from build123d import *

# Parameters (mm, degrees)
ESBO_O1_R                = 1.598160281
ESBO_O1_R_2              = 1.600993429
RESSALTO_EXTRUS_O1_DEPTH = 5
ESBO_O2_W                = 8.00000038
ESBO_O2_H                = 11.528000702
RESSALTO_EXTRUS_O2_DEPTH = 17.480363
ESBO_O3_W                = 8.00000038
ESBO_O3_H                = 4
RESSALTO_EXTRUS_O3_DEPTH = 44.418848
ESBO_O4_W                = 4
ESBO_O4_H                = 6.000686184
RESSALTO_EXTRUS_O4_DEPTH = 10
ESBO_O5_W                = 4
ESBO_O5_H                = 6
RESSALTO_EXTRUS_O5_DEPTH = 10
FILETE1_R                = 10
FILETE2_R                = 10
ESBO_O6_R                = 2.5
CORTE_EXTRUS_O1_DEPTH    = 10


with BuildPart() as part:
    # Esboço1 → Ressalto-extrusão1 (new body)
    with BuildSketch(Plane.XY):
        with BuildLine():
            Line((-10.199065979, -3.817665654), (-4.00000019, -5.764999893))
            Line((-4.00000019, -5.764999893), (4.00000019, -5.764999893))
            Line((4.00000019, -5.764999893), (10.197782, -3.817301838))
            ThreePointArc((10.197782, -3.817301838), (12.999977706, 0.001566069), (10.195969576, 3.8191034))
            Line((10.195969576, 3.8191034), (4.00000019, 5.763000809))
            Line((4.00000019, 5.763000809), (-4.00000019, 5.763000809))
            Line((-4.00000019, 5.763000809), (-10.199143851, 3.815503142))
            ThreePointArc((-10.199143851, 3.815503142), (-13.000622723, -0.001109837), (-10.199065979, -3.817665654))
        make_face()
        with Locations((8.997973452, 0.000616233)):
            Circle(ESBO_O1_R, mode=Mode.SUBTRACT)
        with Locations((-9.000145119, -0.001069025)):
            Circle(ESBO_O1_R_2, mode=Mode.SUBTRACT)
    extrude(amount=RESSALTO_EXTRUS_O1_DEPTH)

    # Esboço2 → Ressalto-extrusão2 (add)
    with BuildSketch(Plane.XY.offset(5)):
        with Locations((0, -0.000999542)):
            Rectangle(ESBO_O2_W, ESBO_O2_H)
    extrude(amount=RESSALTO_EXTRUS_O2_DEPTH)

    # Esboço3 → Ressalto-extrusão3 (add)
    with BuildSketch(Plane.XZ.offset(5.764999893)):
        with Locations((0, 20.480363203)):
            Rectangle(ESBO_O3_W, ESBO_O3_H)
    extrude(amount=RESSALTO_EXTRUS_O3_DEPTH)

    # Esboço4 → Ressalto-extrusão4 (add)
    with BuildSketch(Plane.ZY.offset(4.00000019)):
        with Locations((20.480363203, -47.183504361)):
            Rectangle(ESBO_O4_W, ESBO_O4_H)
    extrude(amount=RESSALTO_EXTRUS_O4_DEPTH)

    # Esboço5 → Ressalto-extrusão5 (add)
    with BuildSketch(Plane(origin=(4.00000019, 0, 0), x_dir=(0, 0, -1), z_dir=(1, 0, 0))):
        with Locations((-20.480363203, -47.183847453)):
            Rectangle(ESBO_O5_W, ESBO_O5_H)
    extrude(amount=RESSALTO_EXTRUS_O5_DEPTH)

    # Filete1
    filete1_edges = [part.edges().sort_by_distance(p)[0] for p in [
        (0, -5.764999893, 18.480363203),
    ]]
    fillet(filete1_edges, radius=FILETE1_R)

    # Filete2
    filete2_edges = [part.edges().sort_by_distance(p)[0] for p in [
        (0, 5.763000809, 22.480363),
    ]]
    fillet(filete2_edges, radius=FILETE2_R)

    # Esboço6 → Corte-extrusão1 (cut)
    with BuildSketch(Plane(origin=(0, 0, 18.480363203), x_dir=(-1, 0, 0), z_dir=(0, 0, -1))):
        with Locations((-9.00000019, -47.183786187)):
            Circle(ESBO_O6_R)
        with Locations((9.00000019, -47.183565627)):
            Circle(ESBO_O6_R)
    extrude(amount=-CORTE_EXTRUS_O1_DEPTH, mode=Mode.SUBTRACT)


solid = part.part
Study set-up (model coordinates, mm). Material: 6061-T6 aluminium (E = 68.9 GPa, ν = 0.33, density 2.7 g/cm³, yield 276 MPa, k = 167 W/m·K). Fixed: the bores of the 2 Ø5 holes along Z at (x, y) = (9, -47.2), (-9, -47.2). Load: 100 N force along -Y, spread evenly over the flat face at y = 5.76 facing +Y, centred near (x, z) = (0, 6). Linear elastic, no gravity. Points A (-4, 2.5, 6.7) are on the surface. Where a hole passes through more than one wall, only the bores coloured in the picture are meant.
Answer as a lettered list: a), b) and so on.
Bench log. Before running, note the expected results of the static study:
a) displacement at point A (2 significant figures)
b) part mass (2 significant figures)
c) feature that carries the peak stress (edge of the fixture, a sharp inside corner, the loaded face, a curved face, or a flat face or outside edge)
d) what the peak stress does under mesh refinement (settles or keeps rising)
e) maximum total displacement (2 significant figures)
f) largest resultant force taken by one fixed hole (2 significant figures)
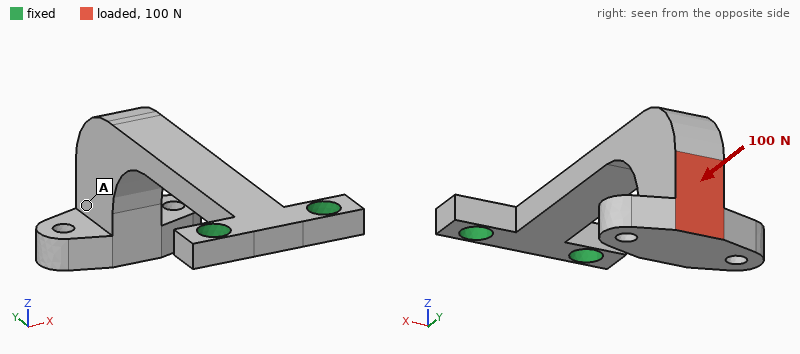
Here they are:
a) 0.65 mm
b) 12 g
c) a sharp inside corner
d) keeps rising
e) 0.76 mm
f) 52 N
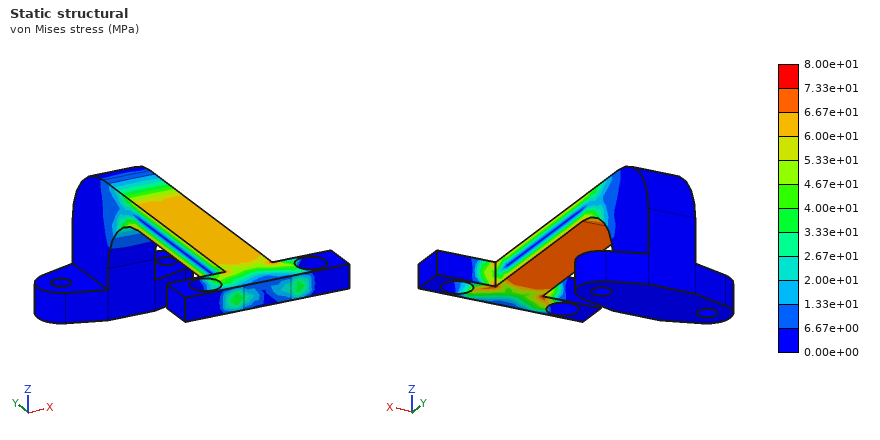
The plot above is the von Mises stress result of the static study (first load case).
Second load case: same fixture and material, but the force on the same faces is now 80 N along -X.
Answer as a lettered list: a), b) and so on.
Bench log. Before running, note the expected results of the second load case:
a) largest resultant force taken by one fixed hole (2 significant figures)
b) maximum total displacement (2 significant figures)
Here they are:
a) 360 N
b) 0.59 mm
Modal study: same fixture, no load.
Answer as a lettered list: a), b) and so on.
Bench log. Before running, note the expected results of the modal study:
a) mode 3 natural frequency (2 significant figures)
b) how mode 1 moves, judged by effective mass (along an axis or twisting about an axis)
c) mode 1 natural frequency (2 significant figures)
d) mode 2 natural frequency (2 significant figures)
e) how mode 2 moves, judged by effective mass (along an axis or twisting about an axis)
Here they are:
a) 2500 Hz
b) along Z
c) 470 Hz
d) 840 Hz
e) along X
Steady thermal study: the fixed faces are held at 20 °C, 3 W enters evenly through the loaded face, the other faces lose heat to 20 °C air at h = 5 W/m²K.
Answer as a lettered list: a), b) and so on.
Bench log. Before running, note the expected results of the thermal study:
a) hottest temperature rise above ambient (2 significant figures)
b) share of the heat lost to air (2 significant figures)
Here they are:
a) 25 K
b) 7.1 %
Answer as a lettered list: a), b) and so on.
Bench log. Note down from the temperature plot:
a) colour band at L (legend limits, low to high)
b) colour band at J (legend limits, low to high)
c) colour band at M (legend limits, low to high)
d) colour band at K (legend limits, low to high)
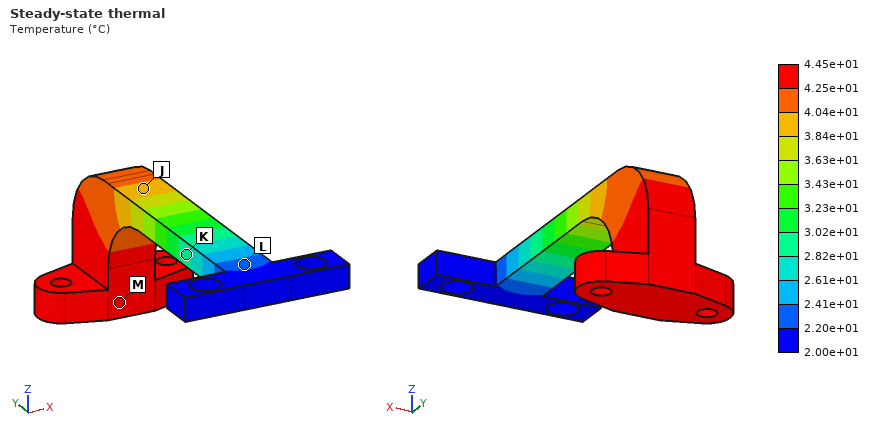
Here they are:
a) 2.20e+01 to 2.41e+01 °C
b) 3.84e+01 to 4.04e+01 °C
c) 4.25e+01 to 4.45e+01 °C
d) 2.82e+01 to 3.02e+01 °C
